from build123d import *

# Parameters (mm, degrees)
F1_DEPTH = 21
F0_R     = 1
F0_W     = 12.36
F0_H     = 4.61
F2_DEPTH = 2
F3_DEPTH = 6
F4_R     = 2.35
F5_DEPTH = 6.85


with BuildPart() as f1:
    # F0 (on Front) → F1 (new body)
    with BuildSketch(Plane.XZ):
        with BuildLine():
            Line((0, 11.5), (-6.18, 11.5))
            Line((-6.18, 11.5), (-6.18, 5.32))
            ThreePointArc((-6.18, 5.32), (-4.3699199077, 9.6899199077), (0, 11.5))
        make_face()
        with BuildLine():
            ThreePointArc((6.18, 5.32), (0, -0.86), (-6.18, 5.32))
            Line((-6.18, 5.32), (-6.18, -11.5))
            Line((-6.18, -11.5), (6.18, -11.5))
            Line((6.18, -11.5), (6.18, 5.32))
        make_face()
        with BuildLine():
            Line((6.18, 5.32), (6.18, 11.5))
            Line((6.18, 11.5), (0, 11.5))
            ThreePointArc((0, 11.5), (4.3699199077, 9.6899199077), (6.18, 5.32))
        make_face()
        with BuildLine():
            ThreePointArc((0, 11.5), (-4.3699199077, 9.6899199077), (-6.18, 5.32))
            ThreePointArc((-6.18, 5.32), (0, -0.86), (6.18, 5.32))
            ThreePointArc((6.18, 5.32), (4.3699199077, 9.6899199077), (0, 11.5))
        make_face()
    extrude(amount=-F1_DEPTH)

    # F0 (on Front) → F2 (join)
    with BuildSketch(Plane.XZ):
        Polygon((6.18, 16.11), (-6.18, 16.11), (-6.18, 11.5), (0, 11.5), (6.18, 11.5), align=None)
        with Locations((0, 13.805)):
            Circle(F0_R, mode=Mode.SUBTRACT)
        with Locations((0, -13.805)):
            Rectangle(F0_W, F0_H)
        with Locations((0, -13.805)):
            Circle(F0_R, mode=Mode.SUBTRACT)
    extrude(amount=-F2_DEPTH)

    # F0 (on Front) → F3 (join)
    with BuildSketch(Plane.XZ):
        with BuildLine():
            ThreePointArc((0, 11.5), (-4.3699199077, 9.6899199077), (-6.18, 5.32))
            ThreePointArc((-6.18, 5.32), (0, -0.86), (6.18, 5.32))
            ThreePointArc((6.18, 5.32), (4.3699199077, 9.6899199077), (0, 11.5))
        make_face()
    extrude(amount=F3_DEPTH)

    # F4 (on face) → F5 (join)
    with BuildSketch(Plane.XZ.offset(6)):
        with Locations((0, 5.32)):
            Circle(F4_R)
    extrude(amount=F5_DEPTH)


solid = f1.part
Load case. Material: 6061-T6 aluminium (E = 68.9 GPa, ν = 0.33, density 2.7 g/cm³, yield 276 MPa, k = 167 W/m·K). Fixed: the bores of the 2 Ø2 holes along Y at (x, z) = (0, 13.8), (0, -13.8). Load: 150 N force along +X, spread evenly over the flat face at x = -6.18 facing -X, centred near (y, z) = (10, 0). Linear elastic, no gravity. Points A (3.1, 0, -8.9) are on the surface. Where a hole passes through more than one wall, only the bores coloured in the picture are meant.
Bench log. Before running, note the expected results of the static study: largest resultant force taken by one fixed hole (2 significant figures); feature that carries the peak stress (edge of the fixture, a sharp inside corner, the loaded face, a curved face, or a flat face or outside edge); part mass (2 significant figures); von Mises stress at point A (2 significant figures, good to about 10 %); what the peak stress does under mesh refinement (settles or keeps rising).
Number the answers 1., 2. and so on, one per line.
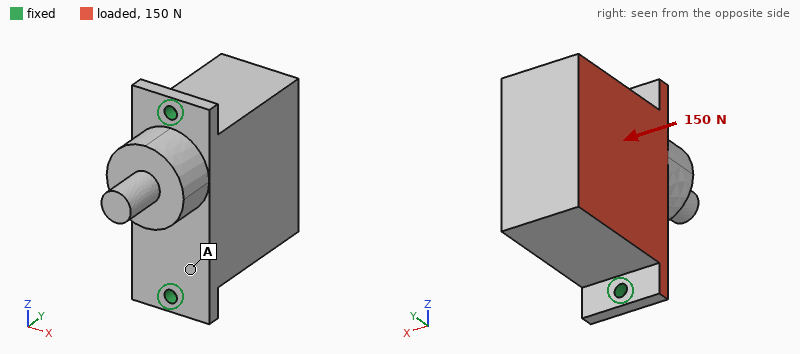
1. 76 N
2. edge of the fixture
3. 19 g
4. 11 MPa
5. keeps rising
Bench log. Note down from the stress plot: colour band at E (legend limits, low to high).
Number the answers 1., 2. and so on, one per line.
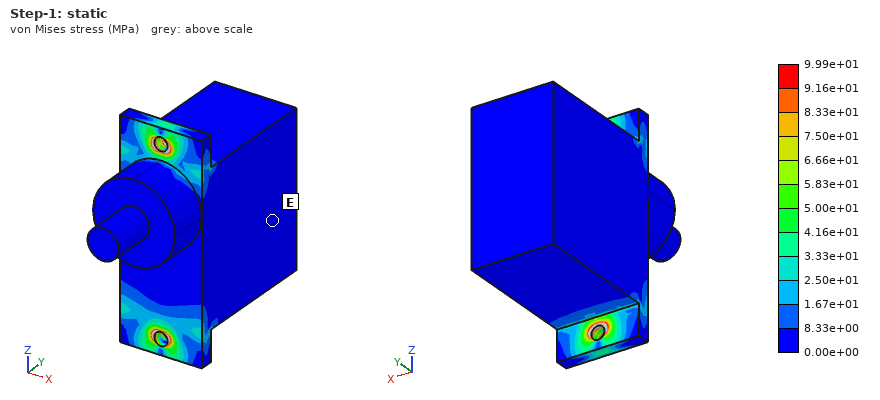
1. 0.00e+00 to 8.33e+00 MPa
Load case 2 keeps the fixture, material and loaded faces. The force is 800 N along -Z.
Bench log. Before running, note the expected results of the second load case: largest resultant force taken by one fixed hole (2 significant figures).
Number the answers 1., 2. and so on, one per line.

1. 530 N
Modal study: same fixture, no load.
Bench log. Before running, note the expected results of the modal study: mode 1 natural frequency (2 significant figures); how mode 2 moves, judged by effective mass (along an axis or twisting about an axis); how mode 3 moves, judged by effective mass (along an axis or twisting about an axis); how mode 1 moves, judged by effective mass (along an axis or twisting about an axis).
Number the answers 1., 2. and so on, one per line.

1. 2400 Hz
2. along Z
3. along Y
4. along X
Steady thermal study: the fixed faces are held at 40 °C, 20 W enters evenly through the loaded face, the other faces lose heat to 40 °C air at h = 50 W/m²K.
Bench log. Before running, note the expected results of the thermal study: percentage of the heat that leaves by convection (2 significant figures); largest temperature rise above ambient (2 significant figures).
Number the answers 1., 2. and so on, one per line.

1. 6.5 %
2. 16 K
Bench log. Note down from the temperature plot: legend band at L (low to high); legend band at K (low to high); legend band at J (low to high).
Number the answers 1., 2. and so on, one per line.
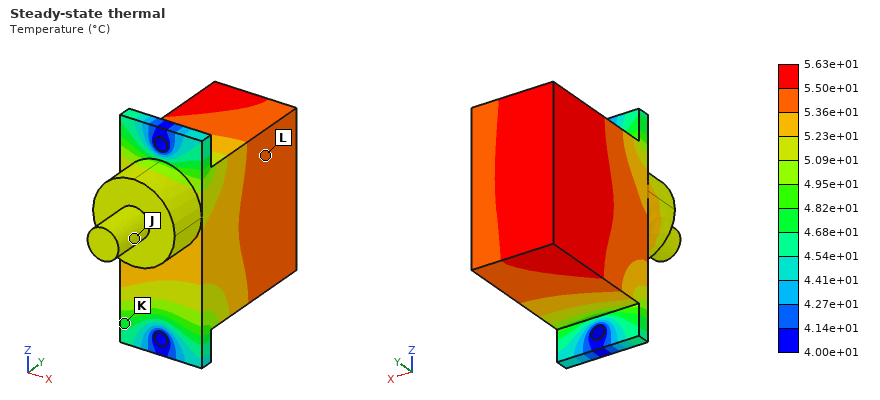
1. 5.36e+01 to 5.50e+01 °C
2. 4.68e+01 to 4.82e+01 °C
3. 5.09e+01 to 5.23e+01 °C
